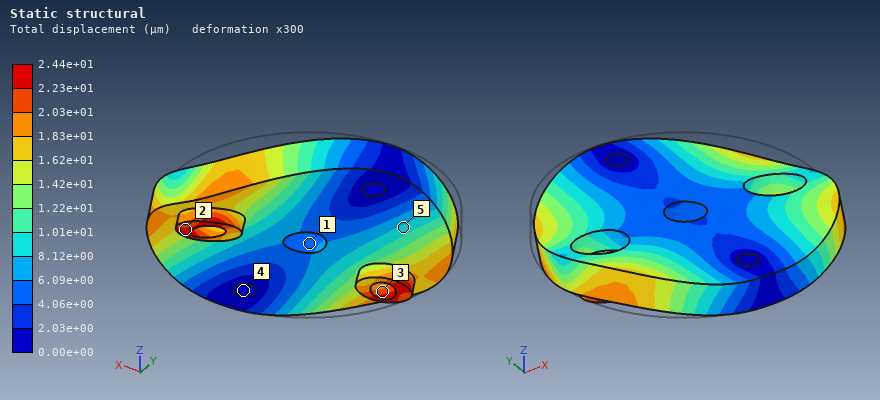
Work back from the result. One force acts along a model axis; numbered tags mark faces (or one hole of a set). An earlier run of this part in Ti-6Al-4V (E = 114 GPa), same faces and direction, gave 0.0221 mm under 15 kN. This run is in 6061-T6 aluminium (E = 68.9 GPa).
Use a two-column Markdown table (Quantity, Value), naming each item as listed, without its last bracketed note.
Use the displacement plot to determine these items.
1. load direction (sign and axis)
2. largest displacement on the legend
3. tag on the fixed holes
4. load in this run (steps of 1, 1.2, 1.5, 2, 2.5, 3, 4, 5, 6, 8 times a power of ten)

| Quantity | Value |
|---|---|
| load direction | -Y |
| largest displacement on the legend | 2.44e+01 µm |
| tag on the fixed holes | 4 |
| load in this run | 10 kN |
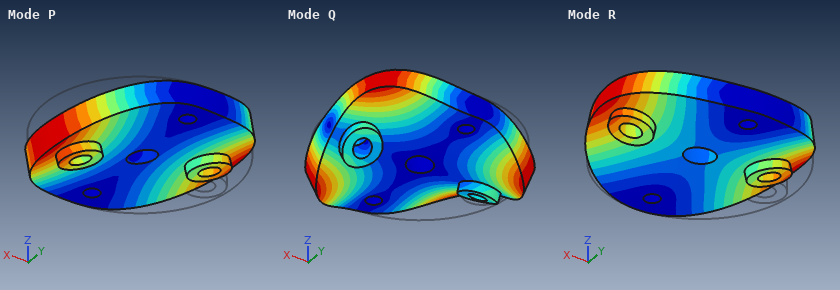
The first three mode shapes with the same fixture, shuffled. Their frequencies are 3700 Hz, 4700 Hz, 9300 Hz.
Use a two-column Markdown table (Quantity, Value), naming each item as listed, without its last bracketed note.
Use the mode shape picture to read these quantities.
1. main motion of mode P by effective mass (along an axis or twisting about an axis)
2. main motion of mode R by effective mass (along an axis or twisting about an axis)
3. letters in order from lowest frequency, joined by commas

| Quantity | Value |
|---|---|
| main motion of mode P by effective mass | twisting about Y |
| main motion of mode R by effective mass | along Z |
| letters in order from lowest frequency, joined by commas | P, R, Q |
